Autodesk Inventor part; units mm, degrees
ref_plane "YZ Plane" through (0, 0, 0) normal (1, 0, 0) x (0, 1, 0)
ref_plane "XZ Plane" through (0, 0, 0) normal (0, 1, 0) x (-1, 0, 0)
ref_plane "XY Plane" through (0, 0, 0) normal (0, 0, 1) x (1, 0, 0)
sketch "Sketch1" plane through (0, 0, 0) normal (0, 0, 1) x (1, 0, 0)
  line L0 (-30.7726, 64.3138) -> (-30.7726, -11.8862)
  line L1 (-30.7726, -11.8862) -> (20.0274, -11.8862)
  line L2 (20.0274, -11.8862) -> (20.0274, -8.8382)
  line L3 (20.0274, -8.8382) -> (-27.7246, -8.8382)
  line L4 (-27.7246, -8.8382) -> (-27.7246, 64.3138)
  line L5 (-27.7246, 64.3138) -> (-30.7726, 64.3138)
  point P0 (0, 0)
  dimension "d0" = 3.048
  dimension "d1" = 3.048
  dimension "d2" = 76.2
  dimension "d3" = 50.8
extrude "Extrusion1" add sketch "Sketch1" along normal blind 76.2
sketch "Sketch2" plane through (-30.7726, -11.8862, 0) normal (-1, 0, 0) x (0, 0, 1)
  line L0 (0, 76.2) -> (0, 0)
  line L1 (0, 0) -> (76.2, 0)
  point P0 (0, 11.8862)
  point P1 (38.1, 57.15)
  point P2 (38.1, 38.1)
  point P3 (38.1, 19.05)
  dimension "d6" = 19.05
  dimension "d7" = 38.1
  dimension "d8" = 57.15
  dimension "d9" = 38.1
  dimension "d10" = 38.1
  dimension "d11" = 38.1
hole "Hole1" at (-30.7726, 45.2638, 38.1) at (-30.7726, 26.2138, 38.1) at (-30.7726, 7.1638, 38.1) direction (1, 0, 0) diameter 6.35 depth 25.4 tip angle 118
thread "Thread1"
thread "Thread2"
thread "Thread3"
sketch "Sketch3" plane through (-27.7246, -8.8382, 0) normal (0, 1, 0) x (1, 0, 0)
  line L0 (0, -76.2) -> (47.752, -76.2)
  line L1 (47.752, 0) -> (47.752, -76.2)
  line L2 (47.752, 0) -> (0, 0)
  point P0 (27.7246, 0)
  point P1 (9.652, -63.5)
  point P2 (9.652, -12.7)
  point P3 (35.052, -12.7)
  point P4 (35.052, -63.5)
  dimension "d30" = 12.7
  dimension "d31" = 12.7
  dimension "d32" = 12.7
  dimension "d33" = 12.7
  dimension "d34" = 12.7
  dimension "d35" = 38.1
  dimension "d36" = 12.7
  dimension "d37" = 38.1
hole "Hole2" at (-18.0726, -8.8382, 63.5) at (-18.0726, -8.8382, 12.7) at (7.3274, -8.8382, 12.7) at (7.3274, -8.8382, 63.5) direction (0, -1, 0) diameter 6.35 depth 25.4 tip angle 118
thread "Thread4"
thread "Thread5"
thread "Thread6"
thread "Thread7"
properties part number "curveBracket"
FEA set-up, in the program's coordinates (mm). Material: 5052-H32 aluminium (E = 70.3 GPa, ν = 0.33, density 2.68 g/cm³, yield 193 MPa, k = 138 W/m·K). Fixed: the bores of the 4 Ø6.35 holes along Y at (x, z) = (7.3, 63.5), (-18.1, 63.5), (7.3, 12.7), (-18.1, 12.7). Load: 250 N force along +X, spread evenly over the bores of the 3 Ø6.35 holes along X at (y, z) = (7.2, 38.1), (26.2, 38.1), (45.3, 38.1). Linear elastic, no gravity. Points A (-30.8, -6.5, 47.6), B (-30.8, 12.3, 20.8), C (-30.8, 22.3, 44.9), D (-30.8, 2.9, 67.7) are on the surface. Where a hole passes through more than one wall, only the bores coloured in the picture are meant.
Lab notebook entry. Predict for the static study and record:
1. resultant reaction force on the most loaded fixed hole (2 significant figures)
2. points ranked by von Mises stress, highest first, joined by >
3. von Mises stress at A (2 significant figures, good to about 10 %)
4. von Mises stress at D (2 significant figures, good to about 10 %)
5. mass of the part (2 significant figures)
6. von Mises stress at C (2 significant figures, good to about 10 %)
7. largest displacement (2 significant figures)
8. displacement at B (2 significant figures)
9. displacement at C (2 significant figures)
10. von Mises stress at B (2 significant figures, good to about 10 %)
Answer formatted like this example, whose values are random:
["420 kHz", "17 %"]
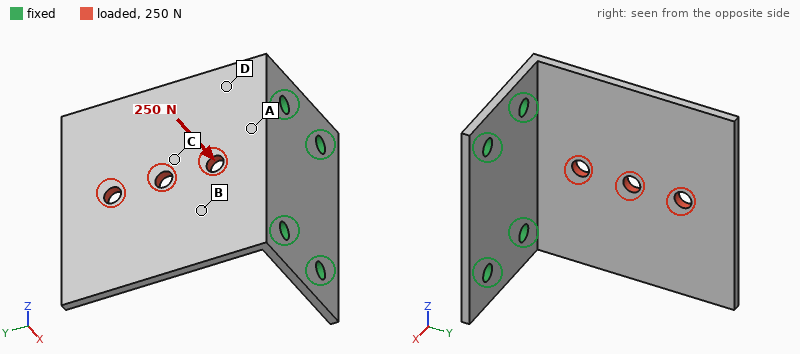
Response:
["98 N", "A > D > B > C", "62 MPa", "50 MPa", "75 g", "18 MPa", "1.4 mm", "0.30 mm", "0.50 mm", "32 MPa"]
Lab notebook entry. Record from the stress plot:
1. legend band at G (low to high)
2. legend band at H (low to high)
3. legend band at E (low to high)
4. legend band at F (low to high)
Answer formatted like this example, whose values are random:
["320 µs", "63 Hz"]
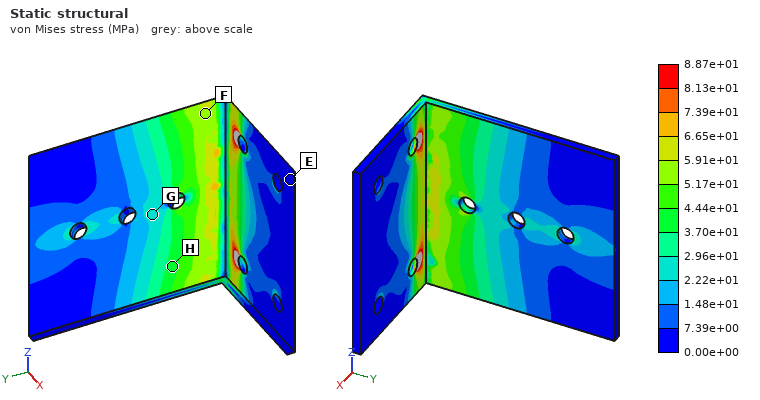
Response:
["2.22e+01 to 2.96e+01 MPa", "3.70e+01 to 4.44e+01 MPa", "0.00e+00 to 7.39e+00 MPa", "5.17e+01 to 5.91e+01 MPa"]
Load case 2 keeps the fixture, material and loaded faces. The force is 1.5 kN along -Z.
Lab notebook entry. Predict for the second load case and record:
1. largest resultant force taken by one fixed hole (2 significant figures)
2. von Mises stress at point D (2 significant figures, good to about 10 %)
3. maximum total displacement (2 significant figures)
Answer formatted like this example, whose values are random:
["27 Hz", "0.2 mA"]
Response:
["1.3 kN", "21 MPa", "0.30 mm"]
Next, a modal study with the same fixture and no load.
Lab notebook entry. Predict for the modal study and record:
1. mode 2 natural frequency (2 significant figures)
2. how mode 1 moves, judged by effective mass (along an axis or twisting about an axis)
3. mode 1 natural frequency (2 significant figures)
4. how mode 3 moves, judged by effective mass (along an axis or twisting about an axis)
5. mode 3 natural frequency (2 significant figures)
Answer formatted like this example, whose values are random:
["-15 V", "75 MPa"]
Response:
["990 Hz", "along X", "380 Hz", "along Z", "2300 Hz"]
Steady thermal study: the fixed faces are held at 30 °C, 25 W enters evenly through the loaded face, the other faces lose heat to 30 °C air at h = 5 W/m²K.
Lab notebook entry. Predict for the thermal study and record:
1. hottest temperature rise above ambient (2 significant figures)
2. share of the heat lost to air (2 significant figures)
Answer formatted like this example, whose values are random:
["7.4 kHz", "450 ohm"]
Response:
["43 K", "7.4 %"]
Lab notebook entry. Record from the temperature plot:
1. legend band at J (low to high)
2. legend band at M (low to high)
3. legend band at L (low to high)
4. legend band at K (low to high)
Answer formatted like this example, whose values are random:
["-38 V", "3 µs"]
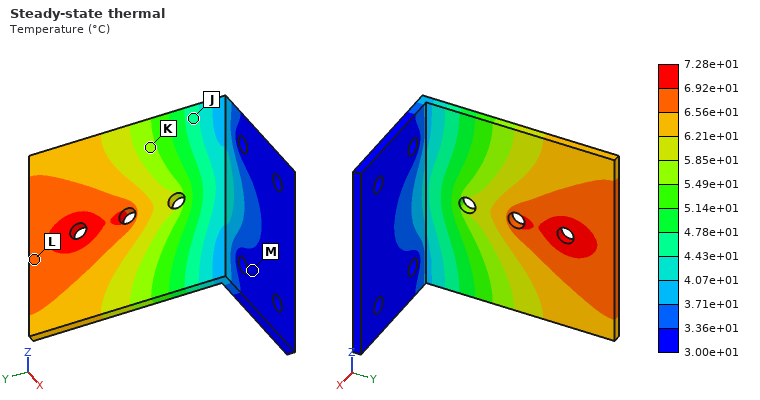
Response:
["4.43e+01 to 4.78e+01 °C", "3.00e+01 to 3.36e+01 °C", "6.56e+01 to 6.92e+01 °C", "5.49e+01 to 5.85e+01 °C"]
